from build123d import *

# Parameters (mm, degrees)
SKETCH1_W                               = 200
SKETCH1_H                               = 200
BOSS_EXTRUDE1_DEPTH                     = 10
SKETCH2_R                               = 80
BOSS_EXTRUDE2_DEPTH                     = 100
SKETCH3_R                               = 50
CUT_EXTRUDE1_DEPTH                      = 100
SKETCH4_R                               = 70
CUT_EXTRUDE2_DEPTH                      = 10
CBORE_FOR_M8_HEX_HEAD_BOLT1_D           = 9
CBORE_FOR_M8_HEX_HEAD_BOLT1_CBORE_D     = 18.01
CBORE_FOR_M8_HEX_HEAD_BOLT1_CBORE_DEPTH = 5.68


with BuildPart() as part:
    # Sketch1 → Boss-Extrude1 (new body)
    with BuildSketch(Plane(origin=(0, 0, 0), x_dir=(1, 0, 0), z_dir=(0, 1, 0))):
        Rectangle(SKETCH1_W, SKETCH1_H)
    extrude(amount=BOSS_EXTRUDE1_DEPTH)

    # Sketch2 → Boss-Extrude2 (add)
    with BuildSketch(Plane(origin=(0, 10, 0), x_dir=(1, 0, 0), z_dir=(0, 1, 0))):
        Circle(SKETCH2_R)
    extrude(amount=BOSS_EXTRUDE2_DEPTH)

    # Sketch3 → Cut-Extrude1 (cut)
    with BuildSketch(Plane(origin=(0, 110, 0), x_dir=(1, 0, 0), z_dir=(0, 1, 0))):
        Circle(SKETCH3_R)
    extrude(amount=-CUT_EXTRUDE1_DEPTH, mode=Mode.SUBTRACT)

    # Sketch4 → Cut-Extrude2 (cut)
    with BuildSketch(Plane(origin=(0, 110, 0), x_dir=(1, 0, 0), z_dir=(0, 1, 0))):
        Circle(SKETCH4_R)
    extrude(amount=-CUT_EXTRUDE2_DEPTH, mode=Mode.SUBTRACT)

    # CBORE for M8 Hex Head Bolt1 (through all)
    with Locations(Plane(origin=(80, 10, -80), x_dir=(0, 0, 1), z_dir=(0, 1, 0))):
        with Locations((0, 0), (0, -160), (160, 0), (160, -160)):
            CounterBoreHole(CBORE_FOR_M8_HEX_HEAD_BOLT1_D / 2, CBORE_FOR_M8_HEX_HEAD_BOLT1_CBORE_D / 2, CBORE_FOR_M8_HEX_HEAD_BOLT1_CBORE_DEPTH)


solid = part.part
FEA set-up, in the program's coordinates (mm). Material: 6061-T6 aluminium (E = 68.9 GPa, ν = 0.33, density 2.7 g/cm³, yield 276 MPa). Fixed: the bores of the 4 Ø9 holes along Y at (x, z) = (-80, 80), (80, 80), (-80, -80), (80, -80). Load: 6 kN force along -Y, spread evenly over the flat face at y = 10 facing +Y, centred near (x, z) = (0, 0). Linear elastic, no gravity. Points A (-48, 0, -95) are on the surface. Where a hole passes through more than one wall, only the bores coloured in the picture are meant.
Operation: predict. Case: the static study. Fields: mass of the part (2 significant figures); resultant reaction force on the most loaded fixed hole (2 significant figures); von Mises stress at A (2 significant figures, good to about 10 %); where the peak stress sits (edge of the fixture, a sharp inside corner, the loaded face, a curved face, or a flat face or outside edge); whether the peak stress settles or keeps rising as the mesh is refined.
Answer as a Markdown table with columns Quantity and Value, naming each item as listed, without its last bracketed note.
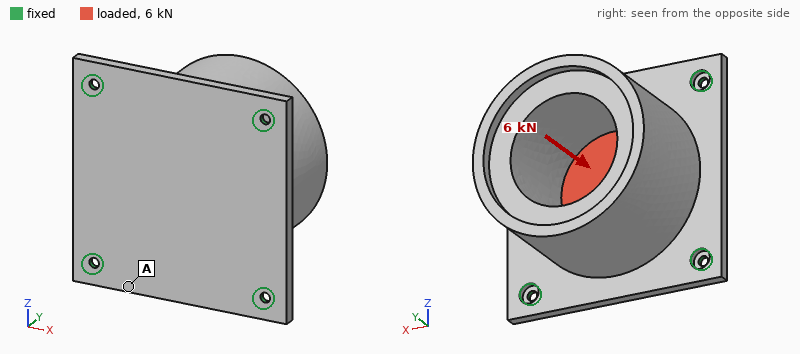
| Quantity | Value |
|---|---|
| mass of the part | 4.2 kg |
| resultant reaction force on the most loaded fixed hole | 2.6 kN |
| von Mises stress at A | 6.6 MPa |
| where the peak stress sits | edge of the fixture |
| whether the peak stress settles or keeps rising as the mesh is refined | keeps rising |
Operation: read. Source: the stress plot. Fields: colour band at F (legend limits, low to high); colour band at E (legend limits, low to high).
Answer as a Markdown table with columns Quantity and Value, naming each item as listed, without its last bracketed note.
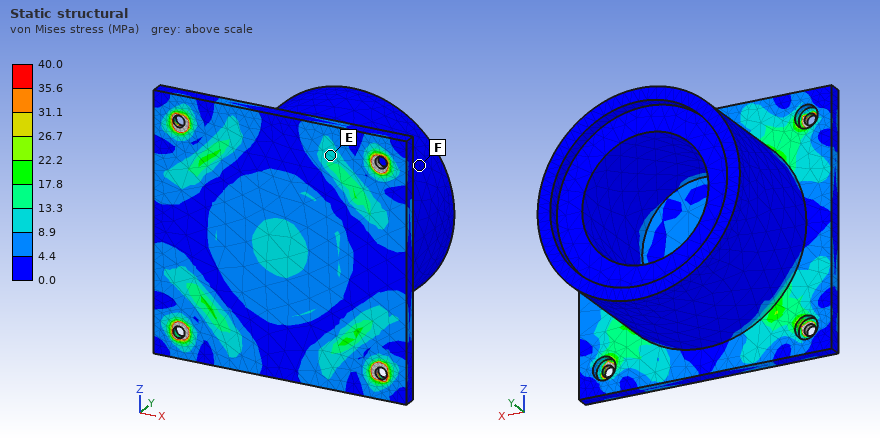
| Quantity | Value |
|---|---|
| colour band at F | 0.0 to 4.4 MPa |
| colour band at E | 8.9 to 13.3 MPa |
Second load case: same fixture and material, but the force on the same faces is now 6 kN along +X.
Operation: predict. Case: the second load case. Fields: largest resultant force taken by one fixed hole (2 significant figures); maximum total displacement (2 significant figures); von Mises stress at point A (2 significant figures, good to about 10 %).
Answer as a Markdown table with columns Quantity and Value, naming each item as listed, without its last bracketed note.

| Quantity | Value |
|---|---|
| largest resultant force taken by one fixed hole | 1.6 kN |
| maximum total displacement | 6.5 µm |
| von Mises stress at point A | 2.5 MPa |
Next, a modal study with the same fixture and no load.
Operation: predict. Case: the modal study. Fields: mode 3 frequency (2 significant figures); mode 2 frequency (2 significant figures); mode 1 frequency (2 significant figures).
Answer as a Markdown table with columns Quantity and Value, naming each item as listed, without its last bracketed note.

| Quantity | Value |
|---|---|
| mode 3 frequency | 990 Hz |
| mode 2 frequency | 980 Hz |
| mode 1 frequency | 960 Hz |
